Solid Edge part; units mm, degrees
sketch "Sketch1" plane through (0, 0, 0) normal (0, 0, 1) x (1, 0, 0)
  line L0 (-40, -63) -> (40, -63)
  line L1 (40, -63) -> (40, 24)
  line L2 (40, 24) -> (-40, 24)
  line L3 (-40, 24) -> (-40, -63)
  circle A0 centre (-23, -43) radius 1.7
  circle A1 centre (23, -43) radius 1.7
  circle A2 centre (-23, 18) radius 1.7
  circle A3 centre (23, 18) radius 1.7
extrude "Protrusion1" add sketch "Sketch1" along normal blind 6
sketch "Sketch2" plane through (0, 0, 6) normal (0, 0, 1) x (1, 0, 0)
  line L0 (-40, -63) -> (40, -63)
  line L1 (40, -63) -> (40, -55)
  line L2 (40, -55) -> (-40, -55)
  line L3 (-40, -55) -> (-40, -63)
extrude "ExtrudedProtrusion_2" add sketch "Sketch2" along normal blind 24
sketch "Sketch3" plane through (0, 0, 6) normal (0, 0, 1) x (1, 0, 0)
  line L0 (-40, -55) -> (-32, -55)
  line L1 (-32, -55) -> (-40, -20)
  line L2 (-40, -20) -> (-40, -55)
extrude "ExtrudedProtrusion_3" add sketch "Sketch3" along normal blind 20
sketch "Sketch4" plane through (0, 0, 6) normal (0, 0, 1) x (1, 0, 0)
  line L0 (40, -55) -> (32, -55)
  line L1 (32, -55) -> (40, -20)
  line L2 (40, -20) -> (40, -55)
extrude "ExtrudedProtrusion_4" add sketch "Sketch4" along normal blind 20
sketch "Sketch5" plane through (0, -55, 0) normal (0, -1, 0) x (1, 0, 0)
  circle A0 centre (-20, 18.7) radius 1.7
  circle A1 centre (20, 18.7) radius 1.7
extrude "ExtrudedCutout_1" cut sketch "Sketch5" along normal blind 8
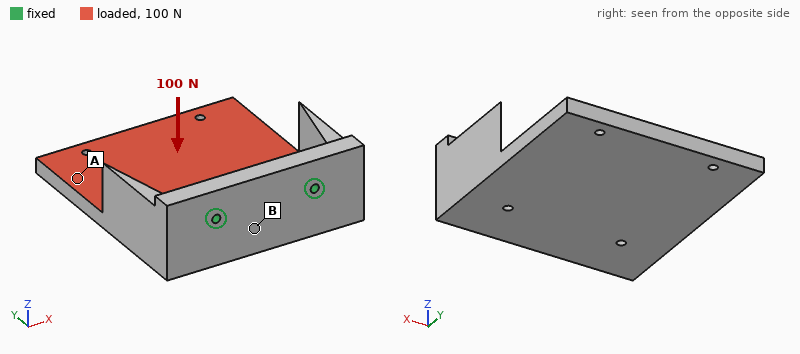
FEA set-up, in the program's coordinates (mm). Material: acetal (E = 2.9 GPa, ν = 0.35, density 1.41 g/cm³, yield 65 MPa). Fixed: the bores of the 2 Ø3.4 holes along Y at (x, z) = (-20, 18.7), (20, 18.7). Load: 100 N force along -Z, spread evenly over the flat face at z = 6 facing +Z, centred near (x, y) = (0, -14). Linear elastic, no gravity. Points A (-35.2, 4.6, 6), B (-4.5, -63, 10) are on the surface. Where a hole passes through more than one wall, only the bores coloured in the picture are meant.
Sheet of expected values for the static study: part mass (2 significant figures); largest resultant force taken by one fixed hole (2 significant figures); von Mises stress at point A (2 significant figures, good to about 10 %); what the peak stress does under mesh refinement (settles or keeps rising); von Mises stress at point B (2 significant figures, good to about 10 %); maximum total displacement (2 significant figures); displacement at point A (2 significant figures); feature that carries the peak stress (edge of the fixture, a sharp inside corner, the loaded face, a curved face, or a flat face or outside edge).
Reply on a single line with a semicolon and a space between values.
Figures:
88 g; 50 N; 1.0 MPa; keeps rising; 2.3 MPa; 1.4 mm; 0.86 mm; edge of the fixture
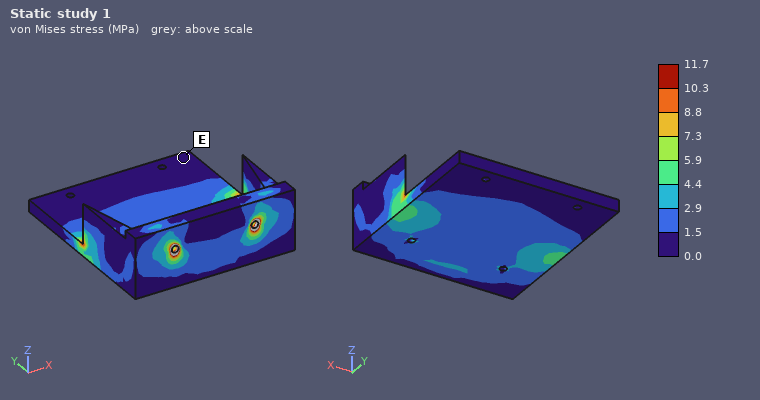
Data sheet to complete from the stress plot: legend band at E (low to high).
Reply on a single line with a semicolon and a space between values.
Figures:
0.0 to 1.5 MPa
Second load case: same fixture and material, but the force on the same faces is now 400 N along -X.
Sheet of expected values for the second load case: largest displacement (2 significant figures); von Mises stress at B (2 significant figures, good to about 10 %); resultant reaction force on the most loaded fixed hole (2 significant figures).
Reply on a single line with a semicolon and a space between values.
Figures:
0.95 mm; 4.6 MPa; 440 N
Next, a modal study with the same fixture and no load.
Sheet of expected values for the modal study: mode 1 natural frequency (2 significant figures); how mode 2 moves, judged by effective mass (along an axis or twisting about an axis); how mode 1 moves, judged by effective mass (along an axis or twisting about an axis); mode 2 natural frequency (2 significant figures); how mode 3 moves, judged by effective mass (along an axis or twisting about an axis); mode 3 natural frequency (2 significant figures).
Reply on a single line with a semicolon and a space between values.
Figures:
240 Hz; along X; along Z; 510 Hz; along X; 810 Hz
